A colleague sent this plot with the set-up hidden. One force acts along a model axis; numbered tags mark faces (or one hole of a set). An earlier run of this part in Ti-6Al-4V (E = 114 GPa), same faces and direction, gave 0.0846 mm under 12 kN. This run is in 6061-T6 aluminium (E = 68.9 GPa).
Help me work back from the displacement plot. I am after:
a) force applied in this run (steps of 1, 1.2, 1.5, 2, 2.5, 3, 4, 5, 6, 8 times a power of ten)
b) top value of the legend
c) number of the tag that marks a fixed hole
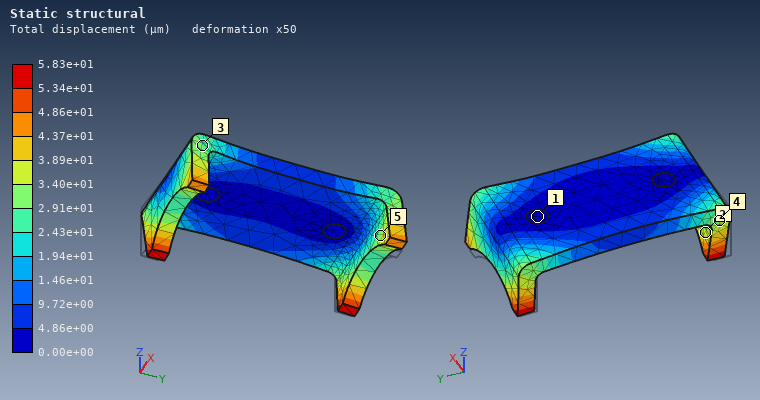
5 kN
5.83e+01 µm
1
